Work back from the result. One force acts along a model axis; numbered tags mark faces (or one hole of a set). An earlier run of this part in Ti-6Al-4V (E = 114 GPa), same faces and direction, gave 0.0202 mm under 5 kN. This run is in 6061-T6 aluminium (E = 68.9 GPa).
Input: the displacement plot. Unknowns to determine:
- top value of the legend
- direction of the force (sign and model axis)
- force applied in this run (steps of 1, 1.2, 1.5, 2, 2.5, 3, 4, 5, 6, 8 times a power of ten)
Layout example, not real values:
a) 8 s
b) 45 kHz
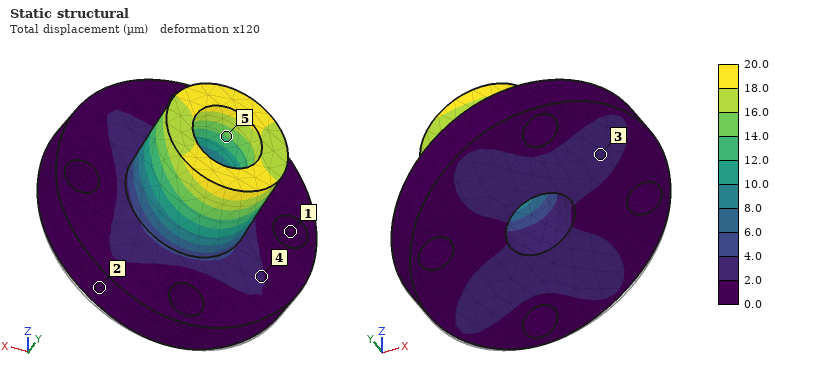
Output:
a) 20.0 µm
b) +Z
c) 3 kN
